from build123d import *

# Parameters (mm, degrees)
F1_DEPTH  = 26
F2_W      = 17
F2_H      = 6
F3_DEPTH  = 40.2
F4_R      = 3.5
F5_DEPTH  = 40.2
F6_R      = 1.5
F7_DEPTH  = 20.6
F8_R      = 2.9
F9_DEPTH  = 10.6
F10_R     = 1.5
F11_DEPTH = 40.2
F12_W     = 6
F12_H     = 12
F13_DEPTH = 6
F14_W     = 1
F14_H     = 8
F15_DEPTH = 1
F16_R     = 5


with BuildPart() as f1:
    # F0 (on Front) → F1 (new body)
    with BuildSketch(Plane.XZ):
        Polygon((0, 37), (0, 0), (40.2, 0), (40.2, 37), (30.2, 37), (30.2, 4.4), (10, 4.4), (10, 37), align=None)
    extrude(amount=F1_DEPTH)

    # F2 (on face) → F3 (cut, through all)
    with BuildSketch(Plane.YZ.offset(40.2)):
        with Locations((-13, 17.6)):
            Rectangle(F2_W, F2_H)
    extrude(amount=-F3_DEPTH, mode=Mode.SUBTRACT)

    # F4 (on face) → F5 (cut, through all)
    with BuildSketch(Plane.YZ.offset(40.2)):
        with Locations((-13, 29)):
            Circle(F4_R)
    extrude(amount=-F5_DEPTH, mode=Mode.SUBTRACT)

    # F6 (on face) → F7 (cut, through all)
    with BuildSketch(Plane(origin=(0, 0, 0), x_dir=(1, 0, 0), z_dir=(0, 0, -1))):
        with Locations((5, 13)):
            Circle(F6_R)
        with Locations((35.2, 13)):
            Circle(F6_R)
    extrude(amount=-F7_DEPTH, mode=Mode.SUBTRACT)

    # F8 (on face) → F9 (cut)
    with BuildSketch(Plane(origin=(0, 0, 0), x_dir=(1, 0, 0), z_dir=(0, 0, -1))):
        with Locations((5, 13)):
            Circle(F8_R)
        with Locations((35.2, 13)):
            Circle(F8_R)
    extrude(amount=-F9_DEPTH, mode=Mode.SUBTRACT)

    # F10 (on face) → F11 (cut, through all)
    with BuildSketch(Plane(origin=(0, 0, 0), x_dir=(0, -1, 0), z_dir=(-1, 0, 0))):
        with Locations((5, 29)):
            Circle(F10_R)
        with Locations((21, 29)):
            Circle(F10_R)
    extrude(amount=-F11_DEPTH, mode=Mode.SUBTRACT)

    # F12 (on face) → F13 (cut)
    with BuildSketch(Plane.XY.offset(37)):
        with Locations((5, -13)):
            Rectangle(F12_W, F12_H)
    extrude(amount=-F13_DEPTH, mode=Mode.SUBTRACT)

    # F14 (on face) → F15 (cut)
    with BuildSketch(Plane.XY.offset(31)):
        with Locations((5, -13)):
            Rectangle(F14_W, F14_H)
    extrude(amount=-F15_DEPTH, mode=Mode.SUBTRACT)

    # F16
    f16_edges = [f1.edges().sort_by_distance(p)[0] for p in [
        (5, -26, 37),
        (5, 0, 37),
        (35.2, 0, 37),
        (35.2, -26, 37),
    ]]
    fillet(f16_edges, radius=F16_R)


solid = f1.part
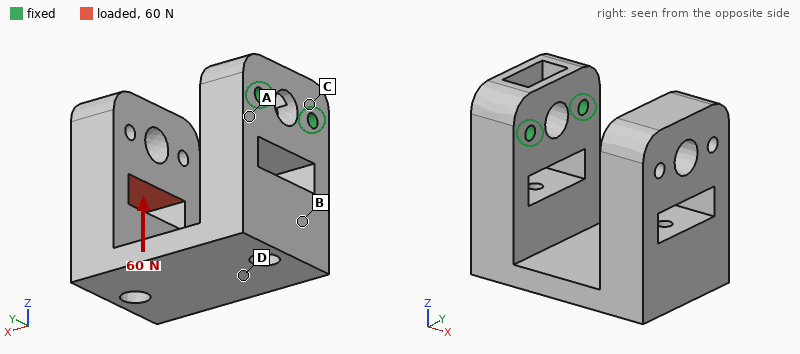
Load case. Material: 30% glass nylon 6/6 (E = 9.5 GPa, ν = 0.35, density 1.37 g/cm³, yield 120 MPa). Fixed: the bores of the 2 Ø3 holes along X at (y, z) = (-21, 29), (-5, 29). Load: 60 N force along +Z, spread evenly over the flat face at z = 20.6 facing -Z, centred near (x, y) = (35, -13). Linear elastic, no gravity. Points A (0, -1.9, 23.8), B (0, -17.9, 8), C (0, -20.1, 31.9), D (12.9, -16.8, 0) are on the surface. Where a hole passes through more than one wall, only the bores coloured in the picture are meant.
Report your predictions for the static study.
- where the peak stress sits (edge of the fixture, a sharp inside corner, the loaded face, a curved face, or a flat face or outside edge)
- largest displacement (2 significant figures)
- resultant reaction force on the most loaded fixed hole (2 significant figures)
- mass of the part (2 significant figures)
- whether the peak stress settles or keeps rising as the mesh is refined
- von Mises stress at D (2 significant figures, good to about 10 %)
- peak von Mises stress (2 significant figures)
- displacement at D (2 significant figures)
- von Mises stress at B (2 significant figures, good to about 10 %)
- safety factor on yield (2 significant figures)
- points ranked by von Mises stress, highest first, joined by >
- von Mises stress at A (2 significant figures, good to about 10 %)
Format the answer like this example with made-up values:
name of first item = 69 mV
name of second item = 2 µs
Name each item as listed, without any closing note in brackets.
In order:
where the peak stress sits = a flat face or outside edge
largest displacement = 0.70 mm
resultant reaction force on the most loaded fixed hole = 30 N
mass of the part = 24 g
whether the peak stress settles or keeps rising as the mesh is refined = settles
von Mises stress at D = 14 MPa
peak von Mises stress = 17 MPa
displacement at D = 0.11 mm
von Mises stress at B = 2.7 MPa
safety factor on yield = 7.0
points ranked by von Mises stress, highest first, joined by > = D > A > B > C
von Mises stress at A = 8.2 MPa
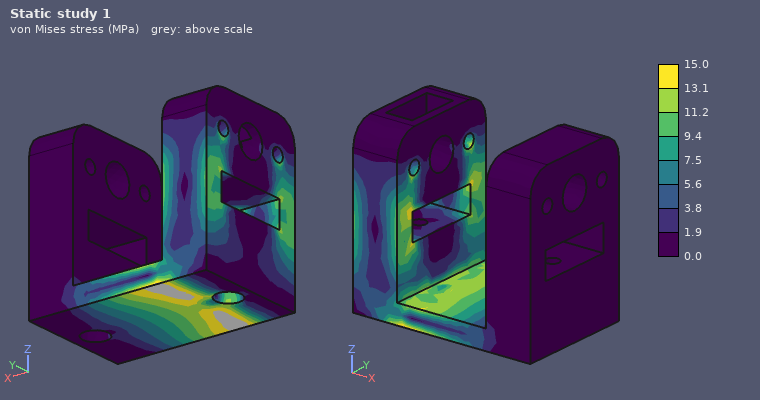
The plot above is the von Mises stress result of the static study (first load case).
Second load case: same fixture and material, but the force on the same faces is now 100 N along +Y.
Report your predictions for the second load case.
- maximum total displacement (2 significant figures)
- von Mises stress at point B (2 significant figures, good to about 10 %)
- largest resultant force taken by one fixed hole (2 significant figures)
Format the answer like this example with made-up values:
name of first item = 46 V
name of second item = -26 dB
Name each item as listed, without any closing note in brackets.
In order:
maximum total displacement = 0.70 mm
von Mises stress at point B = 9.8 MPa
largest resultant force taken by one fixed hole = 130 N
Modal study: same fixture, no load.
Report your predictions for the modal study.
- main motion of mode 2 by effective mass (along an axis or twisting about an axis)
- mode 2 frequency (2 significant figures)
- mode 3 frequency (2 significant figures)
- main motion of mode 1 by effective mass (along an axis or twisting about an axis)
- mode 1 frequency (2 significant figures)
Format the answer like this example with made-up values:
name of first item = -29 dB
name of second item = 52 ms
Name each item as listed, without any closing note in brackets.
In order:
main motion of mode 2 by effective mass = along Y
mode 2 frequency = 720 Hz
mode 3 frequency = 1100 Hz
main motion of mode 1 by effective mass = along Z
mode 1 frequency = 470 Hz
